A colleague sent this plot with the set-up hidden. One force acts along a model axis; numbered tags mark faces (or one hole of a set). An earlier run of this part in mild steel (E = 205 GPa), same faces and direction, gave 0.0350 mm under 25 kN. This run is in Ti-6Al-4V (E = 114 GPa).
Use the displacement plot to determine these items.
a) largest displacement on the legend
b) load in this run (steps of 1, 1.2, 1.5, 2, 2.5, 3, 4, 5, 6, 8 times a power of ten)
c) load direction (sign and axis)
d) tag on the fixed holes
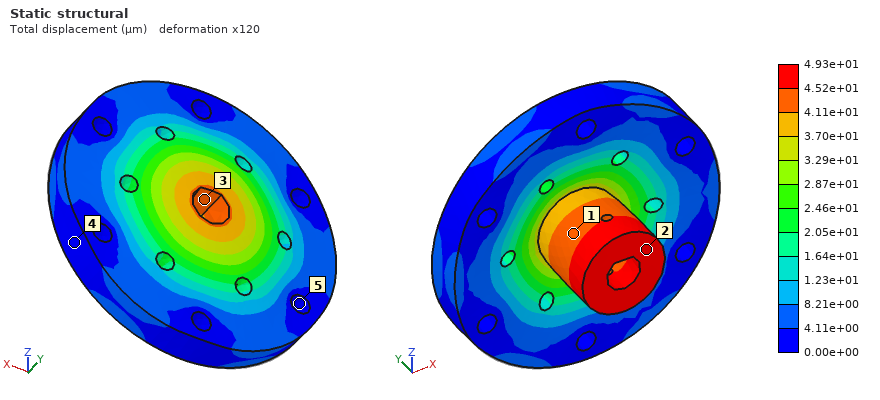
4.93e+01 µm
20 kN
+Y
5
